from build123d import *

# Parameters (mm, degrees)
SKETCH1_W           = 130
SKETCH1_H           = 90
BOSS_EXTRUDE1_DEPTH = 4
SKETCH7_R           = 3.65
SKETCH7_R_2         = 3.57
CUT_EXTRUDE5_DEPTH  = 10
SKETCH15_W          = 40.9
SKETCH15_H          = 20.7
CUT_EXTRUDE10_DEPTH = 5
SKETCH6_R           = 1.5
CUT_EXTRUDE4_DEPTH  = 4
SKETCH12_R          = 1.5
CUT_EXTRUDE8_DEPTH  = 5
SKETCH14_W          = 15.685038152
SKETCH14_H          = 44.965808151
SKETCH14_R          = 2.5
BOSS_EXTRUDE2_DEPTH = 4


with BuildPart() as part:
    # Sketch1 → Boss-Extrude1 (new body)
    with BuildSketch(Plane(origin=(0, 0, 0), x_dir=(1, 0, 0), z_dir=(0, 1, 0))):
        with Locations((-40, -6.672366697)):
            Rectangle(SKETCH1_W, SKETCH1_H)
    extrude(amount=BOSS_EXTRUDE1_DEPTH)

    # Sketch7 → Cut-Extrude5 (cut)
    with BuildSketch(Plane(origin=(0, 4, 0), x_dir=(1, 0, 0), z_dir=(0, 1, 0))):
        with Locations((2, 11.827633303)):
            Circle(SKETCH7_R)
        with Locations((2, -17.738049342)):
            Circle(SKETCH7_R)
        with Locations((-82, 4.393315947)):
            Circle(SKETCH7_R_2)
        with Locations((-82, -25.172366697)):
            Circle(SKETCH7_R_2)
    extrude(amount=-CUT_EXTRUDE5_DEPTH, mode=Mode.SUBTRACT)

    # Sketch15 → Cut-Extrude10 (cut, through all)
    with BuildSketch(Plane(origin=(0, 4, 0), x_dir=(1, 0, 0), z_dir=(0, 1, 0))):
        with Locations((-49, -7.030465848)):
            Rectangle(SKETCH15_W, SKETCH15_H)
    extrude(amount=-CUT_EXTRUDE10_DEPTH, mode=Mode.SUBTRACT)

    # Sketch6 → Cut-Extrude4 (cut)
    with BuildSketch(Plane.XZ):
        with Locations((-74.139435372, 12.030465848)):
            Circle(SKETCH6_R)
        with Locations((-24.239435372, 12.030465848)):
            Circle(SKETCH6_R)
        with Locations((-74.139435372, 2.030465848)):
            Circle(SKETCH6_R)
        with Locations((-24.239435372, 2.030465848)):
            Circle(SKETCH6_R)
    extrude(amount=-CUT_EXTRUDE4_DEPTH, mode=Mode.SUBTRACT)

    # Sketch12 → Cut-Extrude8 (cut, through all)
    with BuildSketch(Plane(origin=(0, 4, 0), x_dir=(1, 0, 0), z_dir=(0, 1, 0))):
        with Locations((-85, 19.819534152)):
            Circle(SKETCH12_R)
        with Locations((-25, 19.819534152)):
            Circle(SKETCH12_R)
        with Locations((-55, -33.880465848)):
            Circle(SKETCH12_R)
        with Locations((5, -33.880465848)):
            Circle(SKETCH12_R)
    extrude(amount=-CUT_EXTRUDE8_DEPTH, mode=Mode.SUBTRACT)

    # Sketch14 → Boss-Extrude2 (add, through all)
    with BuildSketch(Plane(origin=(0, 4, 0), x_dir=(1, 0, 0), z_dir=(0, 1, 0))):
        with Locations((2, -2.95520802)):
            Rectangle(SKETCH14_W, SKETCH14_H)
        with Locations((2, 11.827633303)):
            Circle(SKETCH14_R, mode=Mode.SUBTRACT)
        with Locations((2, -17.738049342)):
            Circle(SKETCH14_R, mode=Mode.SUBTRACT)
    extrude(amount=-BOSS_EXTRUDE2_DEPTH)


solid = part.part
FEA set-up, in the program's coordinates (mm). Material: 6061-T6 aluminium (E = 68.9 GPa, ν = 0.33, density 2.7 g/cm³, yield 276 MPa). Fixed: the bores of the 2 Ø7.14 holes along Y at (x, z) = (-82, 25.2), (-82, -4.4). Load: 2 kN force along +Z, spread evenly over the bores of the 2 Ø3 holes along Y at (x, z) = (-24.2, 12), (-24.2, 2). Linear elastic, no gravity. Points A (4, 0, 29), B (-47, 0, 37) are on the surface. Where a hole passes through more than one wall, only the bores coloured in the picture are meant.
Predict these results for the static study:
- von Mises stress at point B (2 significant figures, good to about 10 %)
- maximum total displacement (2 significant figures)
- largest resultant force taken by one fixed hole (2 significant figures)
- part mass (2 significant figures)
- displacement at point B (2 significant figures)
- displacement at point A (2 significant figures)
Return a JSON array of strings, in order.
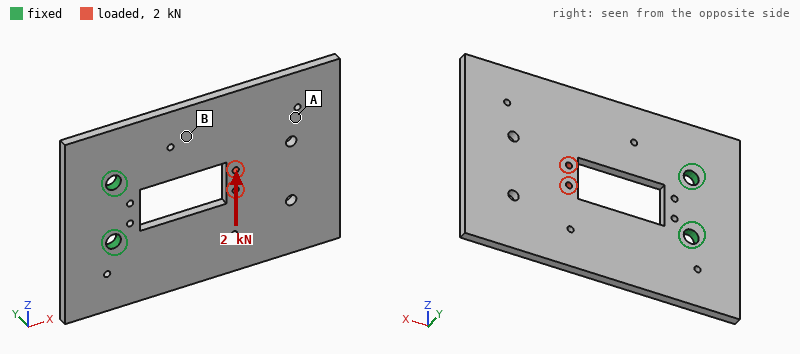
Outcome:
["23 MPa", "0.16 mm", "3.2 kN", "120 g", "0.063 mm", "0.13 mm"]
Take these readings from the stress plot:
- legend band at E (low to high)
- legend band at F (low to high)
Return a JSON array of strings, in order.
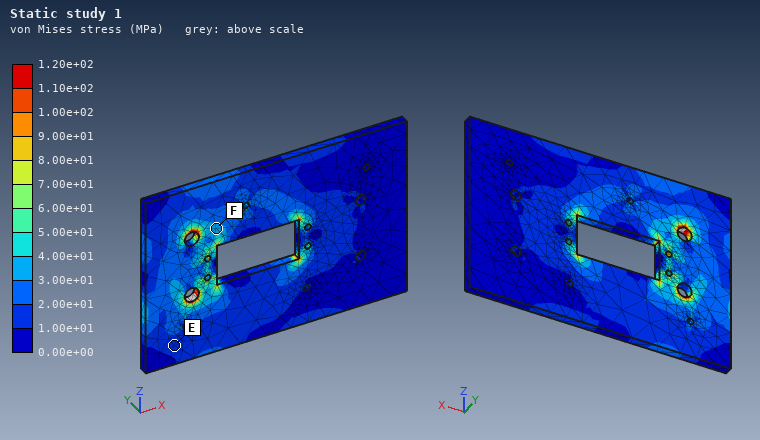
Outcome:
["1.00e+01 to 2.00e+01 MPa", "3.00e+01 to 4.00e+01 MPa"]
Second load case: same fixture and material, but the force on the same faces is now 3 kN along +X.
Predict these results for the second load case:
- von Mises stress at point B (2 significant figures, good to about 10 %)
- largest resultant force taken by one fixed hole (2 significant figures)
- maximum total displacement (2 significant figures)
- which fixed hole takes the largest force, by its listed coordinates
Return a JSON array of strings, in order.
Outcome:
["8.4 MPa", "1.8 kN", "30 µm", "(-82, -4.4)"]
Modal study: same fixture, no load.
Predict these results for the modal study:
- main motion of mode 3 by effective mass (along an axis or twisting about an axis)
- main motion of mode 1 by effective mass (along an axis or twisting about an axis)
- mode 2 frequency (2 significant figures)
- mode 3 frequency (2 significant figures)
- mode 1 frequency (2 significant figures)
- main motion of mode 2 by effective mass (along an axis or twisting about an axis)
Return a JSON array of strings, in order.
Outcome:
["along Y", "along Y", "660 Hz", "1600 Hz", "250 Hz", "twisting about X"]
